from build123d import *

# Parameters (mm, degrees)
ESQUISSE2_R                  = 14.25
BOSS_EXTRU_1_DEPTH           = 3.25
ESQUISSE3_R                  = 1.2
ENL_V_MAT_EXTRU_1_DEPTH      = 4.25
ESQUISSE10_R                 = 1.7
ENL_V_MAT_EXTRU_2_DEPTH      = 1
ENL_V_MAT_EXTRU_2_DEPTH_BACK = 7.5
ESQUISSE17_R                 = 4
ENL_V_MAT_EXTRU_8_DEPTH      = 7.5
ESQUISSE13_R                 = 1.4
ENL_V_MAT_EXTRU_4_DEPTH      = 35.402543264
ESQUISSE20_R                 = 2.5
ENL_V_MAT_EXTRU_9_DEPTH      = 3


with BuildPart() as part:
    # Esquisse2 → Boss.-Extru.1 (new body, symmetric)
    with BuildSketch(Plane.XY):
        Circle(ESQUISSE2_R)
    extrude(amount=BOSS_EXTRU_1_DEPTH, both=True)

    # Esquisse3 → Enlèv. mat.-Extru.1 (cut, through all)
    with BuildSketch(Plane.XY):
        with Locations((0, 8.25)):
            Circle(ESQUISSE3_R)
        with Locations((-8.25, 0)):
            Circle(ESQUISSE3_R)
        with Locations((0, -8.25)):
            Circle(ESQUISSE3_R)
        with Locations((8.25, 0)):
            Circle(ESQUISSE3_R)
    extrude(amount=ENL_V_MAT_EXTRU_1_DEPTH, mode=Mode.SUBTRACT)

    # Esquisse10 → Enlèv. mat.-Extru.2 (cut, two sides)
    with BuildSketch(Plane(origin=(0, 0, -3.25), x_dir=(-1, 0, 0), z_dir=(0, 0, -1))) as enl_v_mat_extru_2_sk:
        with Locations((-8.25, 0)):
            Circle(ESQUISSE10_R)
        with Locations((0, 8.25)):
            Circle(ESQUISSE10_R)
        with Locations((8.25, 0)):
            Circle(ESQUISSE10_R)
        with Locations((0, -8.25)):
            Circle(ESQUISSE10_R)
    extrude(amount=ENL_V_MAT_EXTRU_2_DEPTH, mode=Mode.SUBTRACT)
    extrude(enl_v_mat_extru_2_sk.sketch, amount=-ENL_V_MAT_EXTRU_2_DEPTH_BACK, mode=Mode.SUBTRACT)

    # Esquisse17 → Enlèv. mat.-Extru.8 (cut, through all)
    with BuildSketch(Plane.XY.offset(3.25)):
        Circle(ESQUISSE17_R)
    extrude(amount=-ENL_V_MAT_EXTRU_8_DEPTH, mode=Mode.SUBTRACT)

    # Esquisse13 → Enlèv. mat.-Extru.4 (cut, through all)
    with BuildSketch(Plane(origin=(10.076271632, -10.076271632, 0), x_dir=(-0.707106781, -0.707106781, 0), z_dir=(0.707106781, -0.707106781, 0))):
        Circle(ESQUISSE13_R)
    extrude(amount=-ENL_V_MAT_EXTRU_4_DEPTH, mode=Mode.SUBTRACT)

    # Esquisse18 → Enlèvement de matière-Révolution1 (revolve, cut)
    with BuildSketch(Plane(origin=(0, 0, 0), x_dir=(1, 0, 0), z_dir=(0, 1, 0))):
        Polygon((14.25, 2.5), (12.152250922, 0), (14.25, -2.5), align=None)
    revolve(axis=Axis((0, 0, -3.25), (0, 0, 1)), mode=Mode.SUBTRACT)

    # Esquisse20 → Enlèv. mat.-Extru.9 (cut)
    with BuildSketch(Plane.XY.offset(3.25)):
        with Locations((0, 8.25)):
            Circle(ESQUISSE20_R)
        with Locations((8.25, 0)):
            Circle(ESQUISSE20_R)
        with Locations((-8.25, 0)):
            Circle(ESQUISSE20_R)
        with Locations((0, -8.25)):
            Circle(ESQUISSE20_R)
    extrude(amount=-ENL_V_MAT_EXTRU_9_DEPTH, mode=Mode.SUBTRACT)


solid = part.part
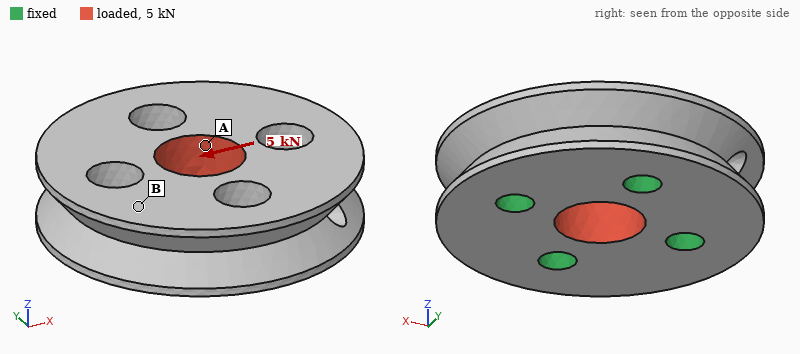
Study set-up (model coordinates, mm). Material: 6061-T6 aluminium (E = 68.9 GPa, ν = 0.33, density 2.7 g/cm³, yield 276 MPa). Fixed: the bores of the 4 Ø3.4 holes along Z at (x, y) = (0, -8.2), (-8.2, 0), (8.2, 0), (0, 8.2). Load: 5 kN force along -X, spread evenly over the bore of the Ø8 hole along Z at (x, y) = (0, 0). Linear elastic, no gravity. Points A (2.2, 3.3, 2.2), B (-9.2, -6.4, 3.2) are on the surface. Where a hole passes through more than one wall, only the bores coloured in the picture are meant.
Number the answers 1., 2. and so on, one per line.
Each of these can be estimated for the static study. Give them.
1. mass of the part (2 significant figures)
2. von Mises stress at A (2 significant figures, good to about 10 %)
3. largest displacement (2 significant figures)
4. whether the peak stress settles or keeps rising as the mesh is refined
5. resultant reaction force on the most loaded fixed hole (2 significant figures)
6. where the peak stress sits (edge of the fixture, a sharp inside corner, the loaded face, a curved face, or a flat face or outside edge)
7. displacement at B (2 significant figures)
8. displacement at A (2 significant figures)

1. 7.8 g
2. 54 MPa
3. 8.1 µm
4. keeps rising
5. 1.4 kN
6. edge of the fixture
7. 4.2 µm
8. 5.3 µm
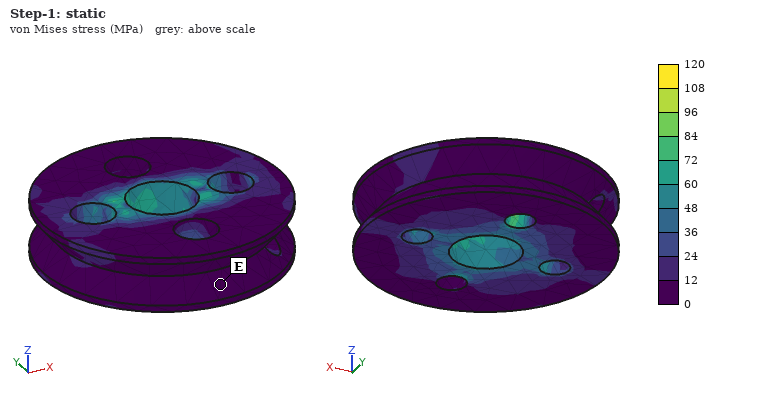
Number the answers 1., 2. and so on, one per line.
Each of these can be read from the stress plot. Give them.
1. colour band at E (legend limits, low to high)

1. 0 to 12 MPa
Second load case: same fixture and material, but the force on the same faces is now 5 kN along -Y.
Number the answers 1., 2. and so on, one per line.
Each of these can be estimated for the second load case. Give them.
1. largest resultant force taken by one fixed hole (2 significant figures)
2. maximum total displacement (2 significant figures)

1. 1.4 kN
2. 8.0 µm
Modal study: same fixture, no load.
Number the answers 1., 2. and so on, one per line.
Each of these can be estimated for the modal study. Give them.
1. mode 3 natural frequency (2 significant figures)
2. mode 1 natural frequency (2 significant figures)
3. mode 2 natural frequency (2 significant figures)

1. 52 kHz
2. 46 kHz
3. 50 kHz
